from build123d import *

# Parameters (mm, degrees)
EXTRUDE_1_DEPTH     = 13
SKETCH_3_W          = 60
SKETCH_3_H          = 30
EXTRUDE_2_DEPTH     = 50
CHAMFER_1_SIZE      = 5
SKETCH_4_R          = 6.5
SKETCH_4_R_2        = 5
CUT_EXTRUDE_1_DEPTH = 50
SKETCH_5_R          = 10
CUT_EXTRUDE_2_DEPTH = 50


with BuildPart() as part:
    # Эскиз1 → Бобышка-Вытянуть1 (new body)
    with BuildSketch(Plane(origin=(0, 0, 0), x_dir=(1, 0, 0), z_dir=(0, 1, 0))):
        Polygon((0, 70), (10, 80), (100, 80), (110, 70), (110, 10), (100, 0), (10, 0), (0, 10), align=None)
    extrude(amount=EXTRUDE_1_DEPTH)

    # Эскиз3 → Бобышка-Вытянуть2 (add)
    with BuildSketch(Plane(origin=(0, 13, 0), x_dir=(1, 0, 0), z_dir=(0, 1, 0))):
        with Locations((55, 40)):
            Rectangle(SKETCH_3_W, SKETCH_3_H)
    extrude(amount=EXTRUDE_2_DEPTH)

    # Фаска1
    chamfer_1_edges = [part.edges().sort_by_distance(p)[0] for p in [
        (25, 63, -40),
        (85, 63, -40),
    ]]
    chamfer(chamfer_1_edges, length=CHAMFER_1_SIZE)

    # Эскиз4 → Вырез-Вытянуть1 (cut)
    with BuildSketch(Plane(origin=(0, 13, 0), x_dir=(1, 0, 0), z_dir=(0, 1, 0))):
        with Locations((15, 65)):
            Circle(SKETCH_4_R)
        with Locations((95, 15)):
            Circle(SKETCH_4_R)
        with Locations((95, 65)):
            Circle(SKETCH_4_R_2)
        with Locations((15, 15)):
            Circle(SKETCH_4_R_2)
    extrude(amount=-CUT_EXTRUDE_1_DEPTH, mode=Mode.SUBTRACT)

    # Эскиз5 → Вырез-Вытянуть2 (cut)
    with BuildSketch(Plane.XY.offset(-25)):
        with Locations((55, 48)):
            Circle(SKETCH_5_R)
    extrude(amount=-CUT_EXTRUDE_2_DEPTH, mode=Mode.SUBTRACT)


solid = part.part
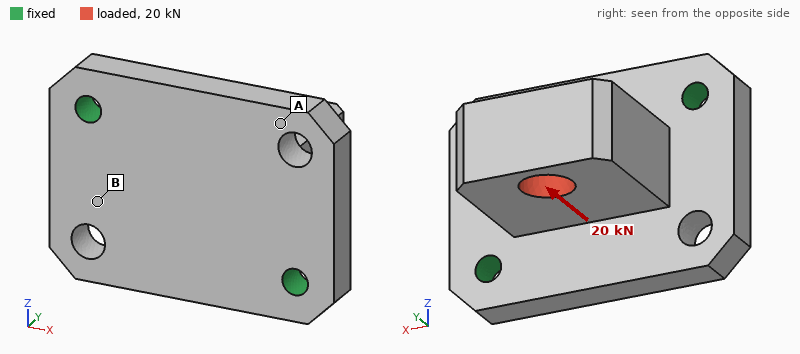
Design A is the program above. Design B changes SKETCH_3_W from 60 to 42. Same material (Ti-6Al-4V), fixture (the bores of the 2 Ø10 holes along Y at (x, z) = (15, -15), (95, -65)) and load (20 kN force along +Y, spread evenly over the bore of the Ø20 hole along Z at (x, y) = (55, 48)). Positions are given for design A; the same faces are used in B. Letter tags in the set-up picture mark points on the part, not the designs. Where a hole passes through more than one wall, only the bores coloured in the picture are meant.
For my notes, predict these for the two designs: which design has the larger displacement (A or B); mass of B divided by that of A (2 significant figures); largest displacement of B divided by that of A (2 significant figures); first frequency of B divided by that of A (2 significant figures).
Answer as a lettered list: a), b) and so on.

a) B
b) 0.85
c) 1.4
d) 1.1
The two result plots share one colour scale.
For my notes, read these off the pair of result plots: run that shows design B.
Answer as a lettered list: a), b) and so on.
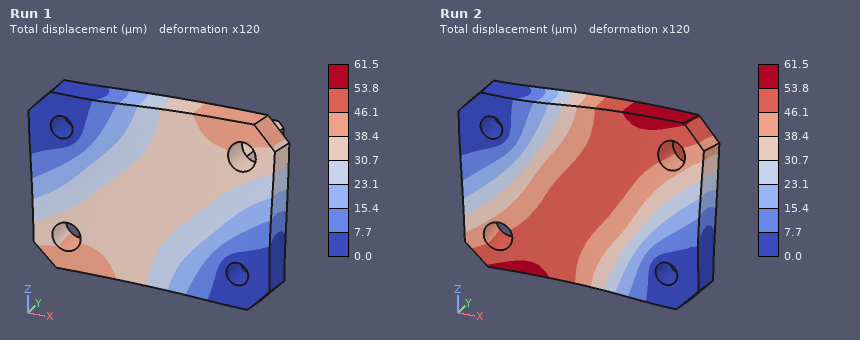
a) Run 2
